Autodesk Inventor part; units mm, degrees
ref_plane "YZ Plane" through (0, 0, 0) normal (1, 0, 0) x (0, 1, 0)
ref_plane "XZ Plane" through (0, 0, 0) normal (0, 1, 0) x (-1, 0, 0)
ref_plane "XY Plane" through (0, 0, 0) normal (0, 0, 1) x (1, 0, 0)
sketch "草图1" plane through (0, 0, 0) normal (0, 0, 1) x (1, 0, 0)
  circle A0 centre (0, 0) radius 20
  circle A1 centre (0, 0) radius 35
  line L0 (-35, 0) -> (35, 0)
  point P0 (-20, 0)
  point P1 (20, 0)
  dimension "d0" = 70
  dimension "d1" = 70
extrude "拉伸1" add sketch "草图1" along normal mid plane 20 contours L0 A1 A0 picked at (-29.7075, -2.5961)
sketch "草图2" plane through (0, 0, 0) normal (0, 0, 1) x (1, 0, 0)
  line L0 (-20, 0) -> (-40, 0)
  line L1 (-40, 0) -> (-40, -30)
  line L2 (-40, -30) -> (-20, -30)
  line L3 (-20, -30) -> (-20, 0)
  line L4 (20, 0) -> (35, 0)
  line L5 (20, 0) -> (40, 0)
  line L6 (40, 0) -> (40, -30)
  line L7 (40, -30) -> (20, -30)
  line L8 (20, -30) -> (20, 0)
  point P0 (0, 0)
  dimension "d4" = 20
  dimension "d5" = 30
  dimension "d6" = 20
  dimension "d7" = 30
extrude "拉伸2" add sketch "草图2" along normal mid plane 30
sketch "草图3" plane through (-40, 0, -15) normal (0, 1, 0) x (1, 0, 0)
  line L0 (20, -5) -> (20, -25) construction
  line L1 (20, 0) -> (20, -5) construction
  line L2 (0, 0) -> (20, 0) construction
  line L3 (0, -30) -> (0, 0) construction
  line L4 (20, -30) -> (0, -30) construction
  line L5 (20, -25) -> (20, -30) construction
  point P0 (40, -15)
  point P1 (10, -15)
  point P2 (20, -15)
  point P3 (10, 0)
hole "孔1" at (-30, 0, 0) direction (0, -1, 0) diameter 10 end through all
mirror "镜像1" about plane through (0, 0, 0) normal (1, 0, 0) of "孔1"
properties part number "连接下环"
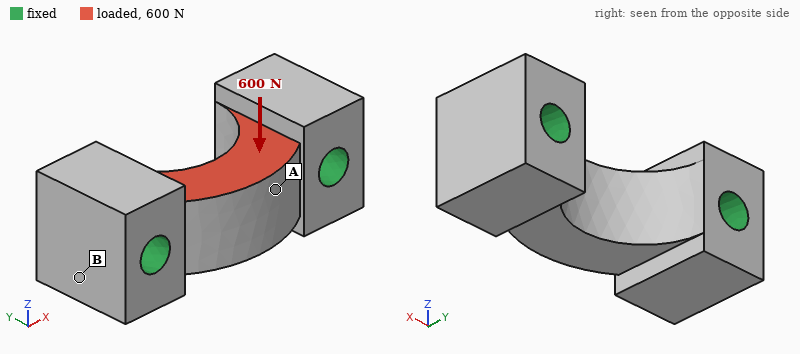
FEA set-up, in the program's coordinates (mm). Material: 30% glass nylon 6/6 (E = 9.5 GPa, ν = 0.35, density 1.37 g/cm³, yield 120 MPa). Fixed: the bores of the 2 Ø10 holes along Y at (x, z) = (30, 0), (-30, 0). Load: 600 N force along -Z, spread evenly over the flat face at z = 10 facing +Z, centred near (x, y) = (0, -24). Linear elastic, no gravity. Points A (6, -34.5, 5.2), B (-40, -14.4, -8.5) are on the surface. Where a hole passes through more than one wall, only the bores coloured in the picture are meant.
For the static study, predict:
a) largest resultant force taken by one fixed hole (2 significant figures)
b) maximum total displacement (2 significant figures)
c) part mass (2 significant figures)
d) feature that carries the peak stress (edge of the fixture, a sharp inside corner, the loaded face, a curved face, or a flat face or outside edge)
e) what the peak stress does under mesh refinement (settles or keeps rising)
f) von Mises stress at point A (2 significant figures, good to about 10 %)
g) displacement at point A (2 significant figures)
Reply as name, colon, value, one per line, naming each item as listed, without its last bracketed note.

largest resultant force taken by one fixed hole: 300 N
maximum total displacement: 11 µm
part mass: 62 g
feature that carries the peak stress: edge of the fixture
what the peak stress does under mesh refinement: keeps rising
von Mises stress at point A: 0.94 MPa
displacement at point A: 10 µm
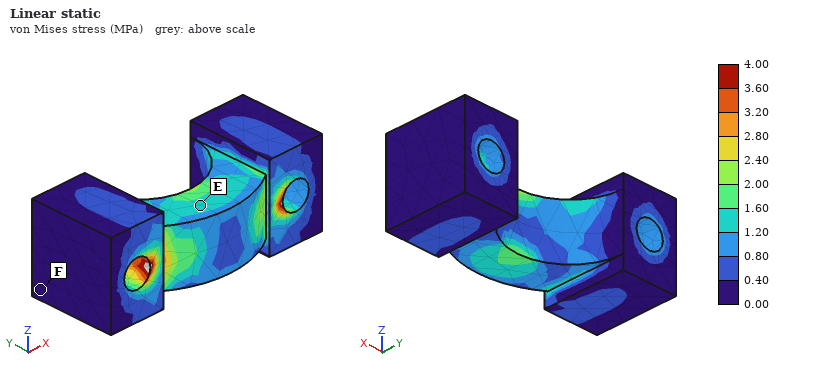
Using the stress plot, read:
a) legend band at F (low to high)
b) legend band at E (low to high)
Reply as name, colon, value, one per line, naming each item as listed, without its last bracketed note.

legend band at F: 0.00 to 0.40 MPa
legend band at E: 1.20 to 1.60 MPa
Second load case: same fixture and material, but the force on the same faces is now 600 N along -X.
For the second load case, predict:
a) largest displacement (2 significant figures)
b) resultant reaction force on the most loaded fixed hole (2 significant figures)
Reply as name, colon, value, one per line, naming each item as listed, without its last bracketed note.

largest displacement: 3.8 µm
resultant reaction force on the most loaded fixed hole: 320 N
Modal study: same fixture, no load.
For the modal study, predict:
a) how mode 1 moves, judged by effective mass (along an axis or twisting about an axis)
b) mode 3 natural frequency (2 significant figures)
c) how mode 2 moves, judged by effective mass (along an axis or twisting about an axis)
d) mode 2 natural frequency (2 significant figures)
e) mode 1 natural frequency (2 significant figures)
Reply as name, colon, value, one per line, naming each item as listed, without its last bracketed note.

how mode 1 moves, judged by effective mass: along Z
mode 3 natural frequency: 18 kHz
how mode 2 moves, judged by effective mass: along Y
mode 2 natural frequency: 14 kHz
mode 1 natural frequency: 10 kHz
